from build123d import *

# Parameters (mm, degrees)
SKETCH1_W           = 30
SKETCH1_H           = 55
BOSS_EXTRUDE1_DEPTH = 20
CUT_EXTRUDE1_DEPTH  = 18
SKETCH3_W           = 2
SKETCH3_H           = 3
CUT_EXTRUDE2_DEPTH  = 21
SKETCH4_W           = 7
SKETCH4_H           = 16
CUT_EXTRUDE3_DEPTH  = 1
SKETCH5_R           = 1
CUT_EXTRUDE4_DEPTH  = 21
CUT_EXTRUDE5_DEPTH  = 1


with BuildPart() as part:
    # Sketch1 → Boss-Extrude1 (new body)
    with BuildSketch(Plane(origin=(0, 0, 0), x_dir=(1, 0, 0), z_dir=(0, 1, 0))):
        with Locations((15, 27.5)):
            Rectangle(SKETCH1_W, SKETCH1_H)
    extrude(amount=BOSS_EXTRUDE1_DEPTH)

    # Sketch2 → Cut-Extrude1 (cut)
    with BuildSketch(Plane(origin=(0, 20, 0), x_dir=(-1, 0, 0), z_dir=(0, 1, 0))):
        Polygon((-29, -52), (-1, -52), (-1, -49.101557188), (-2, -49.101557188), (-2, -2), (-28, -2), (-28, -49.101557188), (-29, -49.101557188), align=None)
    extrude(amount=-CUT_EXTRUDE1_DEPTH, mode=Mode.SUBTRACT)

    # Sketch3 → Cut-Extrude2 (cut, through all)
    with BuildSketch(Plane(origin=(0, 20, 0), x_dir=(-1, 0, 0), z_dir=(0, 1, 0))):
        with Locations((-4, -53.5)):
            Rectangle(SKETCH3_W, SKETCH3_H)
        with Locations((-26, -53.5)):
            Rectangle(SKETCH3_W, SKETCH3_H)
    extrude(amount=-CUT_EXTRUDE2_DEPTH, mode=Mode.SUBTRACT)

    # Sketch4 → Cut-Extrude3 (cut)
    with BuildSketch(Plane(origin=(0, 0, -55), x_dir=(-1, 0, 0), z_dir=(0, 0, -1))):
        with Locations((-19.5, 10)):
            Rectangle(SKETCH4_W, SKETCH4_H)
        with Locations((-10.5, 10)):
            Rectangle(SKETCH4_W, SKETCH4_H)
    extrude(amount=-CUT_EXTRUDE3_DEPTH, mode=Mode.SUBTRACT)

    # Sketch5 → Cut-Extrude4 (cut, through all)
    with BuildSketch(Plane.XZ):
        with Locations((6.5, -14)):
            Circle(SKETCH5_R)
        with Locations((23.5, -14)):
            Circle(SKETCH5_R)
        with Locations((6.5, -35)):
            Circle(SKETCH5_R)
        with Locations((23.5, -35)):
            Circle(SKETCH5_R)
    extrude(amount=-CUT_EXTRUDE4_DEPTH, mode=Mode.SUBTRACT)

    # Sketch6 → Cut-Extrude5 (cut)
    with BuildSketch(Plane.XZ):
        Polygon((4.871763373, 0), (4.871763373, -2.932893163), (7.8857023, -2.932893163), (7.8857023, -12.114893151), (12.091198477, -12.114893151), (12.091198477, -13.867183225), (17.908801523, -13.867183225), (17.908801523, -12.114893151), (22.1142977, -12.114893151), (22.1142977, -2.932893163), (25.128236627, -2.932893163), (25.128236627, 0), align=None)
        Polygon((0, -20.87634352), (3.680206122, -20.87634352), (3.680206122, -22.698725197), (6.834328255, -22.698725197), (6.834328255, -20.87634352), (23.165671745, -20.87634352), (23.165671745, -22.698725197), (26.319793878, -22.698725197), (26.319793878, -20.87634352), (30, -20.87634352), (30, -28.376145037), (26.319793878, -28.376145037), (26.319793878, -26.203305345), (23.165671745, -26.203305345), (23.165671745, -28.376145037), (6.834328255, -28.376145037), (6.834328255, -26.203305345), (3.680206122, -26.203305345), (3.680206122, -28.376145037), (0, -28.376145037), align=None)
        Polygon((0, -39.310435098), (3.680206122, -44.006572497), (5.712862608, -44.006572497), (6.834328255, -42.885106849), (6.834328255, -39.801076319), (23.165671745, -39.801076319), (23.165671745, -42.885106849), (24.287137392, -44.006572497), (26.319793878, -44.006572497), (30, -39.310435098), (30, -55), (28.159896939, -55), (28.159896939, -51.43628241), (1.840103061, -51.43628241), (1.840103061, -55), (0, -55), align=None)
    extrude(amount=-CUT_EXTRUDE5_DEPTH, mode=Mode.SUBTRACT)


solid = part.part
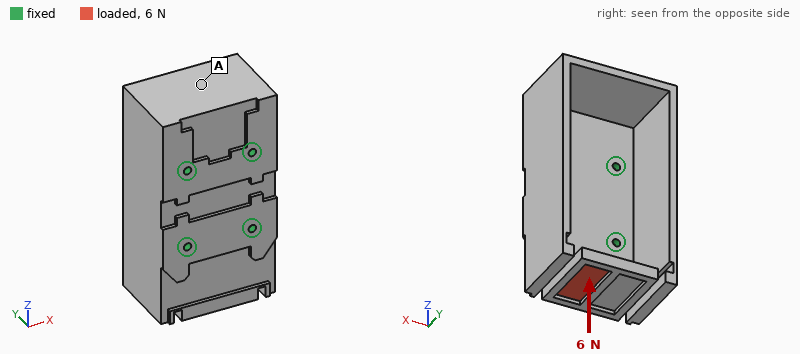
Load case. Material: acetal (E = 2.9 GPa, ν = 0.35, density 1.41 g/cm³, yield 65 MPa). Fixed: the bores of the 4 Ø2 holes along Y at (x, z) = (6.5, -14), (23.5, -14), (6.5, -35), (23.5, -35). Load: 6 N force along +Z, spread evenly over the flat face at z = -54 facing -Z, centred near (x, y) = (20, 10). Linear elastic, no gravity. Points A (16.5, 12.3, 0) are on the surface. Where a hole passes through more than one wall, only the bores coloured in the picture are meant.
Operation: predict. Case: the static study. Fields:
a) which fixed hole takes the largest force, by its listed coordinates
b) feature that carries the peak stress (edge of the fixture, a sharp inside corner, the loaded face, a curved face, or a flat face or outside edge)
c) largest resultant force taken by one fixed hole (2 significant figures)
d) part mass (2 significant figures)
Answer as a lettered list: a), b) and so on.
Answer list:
a) (23.5, -35)
b) a flat face or outside edge
c) 3.7 N
d) 12 g
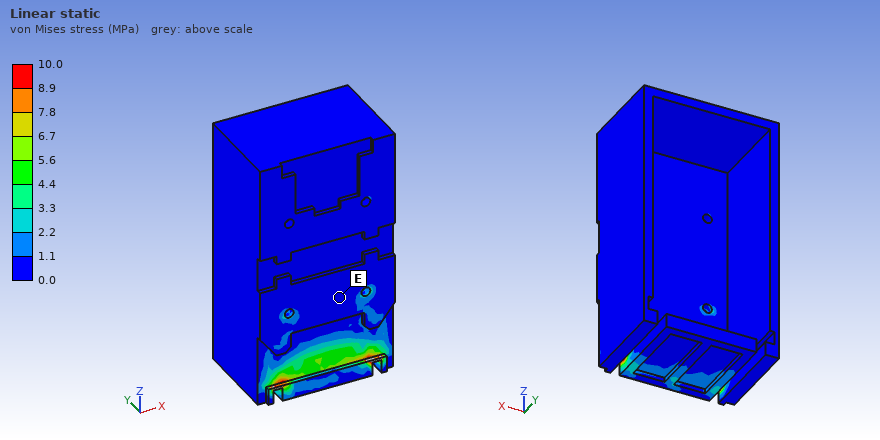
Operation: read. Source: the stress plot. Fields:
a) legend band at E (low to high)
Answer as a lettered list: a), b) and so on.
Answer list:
a) 0.0 to 1.1 MPa
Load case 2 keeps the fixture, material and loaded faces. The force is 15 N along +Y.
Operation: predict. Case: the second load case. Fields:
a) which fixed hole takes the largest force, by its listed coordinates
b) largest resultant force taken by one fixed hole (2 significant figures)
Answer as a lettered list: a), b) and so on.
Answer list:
a) (23.5, -35)
b) 19 N
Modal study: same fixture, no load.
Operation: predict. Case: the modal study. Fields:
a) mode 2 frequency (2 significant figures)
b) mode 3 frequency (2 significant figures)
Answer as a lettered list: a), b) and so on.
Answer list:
a) 830 Hz
b) 850 Hz
